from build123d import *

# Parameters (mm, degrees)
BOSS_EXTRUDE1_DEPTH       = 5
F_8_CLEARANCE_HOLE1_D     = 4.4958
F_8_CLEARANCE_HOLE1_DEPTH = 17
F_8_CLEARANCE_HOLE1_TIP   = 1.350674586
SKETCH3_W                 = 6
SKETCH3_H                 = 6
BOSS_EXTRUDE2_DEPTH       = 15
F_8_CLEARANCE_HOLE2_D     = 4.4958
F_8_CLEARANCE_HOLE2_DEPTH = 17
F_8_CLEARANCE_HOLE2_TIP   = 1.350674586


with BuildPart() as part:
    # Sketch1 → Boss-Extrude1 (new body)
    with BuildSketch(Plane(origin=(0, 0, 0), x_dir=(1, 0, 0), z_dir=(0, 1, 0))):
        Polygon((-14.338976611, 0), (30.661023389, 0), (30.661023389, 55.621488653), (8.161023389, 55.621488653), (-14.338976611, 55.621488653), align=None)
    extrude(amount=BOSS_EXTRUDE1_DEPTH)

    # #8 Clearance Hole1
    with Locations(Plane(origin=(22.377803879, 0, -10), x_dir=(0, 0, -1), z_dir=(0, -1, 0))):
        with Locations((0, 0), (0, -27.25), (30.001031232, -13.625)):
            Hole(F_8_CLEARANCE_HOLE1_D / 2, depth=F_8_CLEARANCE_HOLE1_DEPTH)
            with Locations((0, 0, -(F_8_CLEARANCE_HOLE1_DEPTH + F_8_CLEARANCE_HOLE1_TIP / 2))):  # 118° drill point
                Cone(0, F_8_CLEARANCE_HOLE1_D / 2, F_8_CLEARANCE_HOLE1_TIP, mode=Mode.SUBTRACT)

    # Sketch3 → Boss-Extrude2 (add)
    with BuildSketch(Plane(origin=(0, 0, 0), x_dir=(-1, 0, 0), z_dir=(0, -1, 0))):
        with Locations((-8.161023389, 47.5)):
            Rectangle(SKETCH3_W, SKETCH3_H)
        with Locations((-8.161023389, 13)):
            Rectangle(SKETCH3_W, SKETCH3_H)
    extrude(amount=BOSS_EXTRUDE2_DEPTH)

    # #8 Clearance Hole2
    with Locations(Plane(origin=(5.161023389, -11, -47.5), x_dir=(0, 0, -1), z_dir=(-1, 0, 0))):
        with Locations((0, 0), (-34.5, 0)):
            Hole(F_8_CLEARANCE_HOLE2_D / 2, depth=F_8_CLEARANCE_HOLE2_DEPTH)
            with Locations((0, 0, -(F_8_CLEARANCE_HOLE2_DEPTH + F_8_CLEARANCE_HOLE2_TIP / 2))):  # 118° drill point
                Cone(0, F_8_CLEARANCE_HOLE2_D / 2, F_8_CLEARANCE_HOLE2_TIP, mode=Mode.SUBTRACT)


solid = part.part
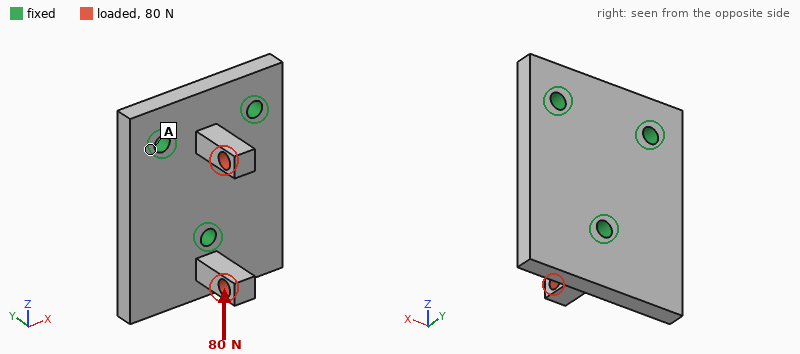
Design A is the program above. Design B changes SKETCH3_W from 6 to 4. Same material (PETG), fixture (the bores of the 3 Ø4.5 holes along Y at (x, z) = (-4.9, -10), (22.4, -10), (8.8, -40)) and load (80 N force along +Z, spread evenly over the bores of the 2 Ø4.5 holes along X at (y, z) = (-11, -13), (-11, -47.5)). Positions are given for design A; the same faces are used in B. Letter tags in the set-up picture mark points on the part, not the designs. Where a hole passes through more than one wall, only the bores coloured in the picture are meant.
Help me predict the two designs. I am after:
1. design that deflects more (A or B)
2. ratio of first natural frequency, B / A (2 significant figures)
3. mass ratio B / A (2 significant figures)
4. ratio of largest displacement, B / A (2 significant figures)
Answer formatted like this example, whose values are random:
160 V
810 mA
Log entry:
B
1.00
0.98
1.3
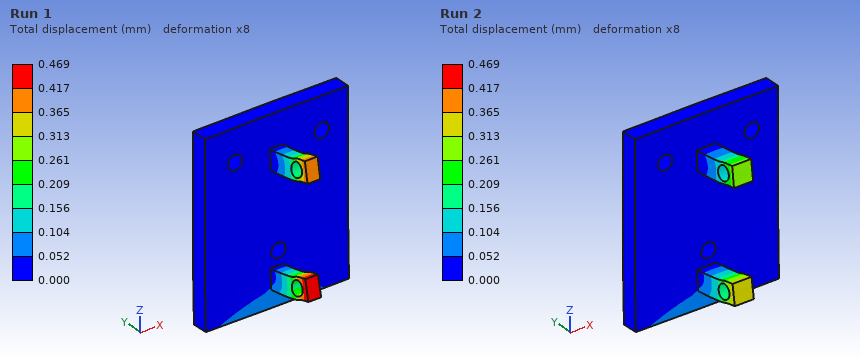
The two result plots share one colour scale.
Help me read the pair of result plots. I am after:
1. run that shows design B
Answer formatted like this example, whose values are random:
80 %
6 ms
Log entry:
Run 1
